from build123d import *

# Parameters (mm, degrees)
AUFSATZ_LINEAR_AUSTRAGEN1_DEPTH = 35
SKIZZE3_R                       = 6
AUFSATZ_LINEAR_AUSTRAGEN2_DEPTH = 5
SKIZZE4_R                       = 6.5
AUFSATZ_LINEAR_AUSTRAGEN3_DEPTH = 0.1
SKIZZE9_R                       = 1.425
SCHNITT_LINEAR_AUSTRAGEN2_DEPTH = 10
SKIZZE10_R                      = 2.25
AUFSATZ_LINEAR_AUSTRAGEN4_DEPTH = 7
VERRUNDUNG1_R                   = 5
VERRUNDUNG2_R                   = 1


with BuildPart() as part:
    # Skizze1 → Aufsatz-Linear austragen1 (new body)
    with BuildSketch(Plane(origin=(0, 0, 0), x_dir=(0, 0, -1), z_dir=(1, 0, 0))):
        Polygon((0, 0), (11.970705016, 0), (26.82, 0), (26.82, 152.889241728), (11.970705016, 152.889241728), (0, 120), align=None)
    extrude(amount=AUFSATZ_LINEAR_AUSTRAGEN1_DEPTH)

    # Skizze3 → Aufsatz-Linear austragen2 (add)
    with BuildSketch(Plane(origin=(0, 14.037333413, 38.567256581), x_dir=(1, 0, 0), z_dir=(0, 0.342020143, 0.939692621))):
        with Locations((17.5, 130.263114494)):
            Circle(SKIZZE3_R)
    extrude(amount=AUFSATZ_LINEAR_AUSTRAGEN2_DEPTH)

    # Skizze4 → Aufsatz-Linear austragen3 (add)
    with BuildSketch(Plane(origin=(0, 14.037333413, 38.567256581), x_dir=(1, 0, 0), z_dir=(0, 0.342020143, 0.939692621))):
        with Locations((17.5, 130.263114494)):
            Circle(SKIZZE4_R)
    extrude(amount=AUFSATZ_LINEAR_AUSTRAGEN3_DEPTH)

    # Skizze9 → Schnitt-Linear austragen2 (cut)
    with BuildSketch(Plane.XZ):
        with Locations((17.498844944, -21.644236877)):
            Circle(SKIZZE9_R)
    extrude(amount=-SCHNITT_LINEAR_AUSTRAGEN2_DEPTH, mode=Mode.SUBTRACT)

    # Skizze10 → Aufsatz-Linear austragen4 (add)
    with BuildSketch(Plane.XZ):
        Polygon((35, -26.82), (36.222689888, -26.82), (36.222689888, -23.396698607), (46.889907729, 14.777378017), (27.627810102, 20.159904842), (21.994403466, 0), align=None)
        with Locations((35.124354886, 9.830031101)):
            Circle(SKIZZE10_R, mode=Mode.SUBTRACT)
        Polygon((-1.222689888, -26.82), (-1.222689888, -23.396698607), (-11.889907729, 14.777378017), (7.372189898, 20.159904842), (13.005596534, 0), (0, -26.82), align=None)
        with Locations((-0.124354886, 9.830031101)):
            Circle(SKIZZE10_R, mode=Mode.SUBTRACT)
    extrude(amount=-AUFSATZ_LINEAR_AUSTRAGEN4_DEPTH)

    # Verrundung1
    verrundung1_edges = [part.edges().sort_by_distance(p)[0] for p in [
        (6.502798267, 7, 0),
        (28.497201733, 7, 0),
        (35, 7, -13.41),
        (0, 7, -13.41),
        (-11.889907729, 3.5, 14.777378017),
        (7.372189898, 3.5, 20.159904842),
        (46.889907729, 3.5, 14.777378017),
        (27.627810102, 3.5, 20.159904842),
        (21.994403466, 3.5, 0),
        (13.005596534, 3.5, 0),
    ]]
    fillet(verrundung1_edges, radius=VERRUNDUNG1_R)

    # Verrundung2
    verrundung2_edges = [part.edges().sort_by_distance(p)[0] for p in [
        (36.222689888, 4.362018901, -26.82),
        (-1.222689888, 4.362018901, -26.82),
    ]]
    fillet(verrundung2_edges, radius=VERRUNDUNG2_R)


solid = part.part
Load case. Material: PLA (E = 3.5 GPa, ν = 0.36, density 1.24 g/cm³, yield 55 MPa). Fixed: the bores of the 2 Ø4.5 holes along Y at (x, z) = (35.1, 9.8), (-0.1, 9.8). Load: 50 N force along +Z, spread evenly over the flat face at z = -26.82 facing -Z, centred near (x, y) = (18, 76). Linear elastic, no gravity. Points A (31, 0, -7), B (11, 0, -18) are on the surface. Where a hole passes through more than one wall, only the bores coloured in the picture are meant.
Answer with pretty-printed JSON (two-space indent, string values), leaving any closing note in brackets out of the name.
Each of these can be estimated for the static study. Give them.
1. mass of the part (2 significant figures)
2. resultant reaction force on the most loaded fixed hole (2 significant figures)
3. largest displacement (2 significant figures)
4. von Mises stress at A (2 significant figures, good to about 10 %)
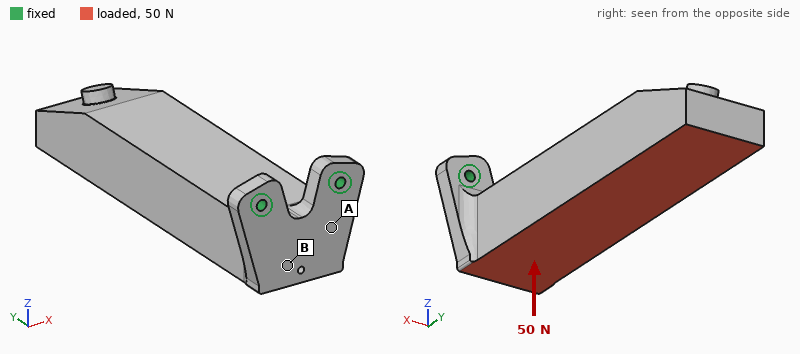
{
  "mass of the part": "180 g",
  "resultant reaction force on the most loaded fixed hole": "29 N",
  "largest displacement": "1.8 mm",
  "von Mises stress at A": "2.7 MPa"
}
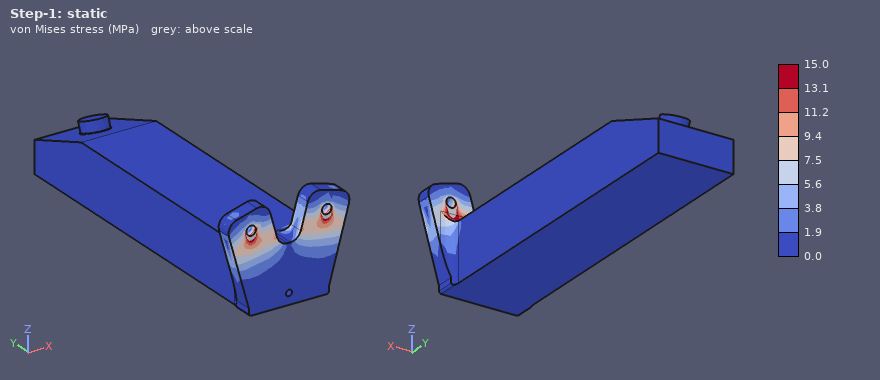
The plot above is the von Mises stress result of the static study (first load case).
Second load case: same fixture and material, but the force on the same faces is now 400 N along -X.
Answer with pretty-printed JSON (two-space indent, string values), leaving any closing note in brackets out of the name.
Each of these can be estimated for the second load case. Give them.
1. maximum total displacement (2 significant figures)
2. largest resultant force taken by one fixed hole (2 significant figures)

{
  "maximum total displacement": "2.0 mm",
  "largest resultant force taken by one fixed hole": "920 N"
}
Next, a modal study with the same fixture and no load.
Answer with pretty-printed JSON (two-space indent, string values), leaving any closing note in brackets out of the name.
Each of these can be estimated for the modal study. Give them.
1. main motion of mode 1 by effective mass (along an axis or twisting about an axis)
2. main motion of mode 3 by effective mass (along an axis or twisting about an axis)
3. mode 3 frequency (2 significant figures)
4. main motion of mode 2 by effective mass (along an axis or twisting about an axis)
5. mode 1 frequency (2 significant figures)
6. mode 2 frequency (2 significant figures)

{
  "main motion of mode 1 by effective mass": "along Z",
  "main motion of mode 3 by effective mass": "along Y",
  "mode 3 frequency": "960 Hz",
  "main motion of mode 2 by effective mass": "along X",
  "mode 1 frequency": "81 Hz",
  "mode 2 frequency": "220 Hz"
}
